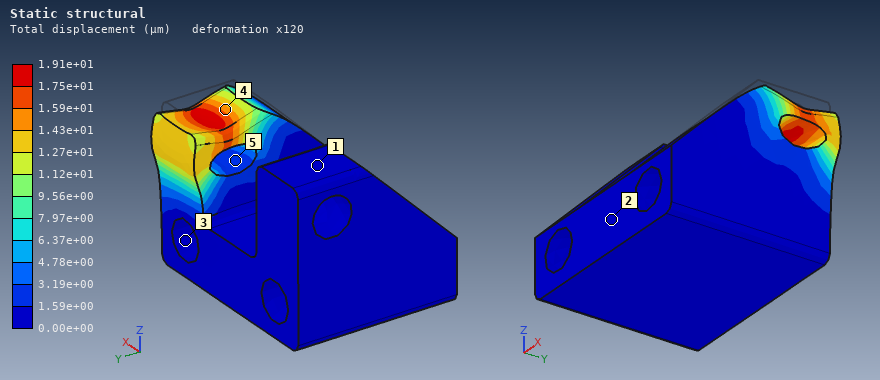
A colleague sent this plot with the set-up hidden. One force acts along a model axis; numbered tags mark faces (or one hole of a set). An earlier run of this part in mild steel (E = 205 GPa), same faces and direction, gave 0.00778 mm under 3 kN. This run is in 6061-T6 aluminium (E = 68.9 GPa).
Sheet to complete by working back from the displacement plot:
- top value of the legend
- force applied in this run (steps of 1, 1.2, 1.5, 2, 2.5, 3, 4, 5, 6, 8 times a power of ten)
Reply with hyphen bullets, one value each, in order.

- 1.91e+01 µm
- 2.5 kN
